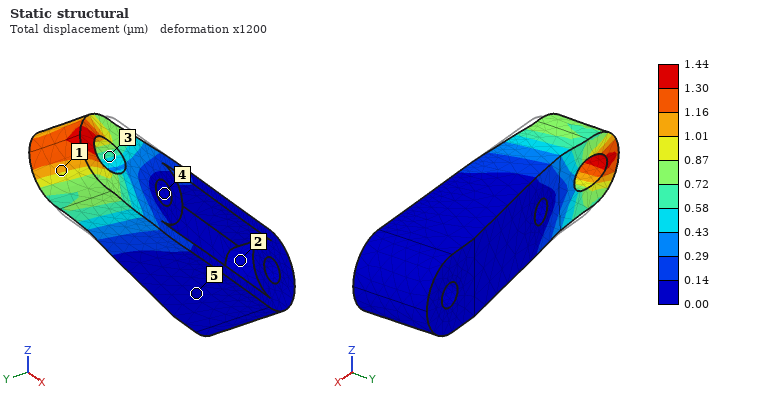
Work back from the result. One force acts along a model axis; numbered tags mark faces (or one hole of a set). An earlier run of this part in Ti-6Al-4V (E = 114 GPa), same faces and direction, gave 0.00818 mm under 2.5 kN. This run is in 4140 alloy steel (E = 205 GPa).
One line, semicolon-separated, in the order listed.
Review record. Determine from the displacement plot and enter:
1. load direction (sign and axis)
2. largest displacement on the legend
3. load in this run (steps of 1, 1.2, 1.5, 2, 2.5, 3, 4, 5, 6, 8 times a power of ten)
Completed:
-X; 1.44 µm; 800 N
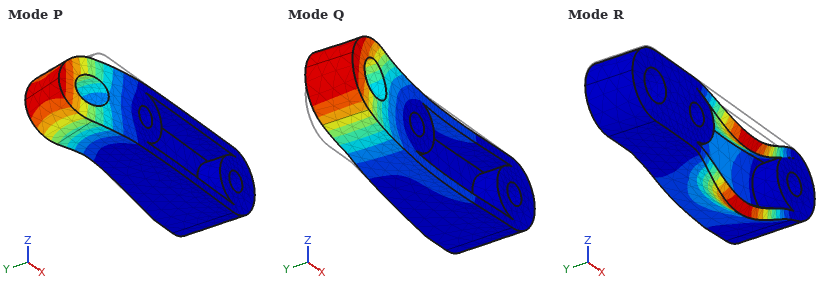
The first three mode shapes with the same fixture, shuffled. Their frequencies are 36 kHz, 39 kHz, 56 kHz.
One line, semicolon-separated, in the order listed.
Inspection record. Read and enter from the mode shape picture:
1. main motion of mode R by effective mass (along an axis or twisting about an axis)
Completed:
along Z
